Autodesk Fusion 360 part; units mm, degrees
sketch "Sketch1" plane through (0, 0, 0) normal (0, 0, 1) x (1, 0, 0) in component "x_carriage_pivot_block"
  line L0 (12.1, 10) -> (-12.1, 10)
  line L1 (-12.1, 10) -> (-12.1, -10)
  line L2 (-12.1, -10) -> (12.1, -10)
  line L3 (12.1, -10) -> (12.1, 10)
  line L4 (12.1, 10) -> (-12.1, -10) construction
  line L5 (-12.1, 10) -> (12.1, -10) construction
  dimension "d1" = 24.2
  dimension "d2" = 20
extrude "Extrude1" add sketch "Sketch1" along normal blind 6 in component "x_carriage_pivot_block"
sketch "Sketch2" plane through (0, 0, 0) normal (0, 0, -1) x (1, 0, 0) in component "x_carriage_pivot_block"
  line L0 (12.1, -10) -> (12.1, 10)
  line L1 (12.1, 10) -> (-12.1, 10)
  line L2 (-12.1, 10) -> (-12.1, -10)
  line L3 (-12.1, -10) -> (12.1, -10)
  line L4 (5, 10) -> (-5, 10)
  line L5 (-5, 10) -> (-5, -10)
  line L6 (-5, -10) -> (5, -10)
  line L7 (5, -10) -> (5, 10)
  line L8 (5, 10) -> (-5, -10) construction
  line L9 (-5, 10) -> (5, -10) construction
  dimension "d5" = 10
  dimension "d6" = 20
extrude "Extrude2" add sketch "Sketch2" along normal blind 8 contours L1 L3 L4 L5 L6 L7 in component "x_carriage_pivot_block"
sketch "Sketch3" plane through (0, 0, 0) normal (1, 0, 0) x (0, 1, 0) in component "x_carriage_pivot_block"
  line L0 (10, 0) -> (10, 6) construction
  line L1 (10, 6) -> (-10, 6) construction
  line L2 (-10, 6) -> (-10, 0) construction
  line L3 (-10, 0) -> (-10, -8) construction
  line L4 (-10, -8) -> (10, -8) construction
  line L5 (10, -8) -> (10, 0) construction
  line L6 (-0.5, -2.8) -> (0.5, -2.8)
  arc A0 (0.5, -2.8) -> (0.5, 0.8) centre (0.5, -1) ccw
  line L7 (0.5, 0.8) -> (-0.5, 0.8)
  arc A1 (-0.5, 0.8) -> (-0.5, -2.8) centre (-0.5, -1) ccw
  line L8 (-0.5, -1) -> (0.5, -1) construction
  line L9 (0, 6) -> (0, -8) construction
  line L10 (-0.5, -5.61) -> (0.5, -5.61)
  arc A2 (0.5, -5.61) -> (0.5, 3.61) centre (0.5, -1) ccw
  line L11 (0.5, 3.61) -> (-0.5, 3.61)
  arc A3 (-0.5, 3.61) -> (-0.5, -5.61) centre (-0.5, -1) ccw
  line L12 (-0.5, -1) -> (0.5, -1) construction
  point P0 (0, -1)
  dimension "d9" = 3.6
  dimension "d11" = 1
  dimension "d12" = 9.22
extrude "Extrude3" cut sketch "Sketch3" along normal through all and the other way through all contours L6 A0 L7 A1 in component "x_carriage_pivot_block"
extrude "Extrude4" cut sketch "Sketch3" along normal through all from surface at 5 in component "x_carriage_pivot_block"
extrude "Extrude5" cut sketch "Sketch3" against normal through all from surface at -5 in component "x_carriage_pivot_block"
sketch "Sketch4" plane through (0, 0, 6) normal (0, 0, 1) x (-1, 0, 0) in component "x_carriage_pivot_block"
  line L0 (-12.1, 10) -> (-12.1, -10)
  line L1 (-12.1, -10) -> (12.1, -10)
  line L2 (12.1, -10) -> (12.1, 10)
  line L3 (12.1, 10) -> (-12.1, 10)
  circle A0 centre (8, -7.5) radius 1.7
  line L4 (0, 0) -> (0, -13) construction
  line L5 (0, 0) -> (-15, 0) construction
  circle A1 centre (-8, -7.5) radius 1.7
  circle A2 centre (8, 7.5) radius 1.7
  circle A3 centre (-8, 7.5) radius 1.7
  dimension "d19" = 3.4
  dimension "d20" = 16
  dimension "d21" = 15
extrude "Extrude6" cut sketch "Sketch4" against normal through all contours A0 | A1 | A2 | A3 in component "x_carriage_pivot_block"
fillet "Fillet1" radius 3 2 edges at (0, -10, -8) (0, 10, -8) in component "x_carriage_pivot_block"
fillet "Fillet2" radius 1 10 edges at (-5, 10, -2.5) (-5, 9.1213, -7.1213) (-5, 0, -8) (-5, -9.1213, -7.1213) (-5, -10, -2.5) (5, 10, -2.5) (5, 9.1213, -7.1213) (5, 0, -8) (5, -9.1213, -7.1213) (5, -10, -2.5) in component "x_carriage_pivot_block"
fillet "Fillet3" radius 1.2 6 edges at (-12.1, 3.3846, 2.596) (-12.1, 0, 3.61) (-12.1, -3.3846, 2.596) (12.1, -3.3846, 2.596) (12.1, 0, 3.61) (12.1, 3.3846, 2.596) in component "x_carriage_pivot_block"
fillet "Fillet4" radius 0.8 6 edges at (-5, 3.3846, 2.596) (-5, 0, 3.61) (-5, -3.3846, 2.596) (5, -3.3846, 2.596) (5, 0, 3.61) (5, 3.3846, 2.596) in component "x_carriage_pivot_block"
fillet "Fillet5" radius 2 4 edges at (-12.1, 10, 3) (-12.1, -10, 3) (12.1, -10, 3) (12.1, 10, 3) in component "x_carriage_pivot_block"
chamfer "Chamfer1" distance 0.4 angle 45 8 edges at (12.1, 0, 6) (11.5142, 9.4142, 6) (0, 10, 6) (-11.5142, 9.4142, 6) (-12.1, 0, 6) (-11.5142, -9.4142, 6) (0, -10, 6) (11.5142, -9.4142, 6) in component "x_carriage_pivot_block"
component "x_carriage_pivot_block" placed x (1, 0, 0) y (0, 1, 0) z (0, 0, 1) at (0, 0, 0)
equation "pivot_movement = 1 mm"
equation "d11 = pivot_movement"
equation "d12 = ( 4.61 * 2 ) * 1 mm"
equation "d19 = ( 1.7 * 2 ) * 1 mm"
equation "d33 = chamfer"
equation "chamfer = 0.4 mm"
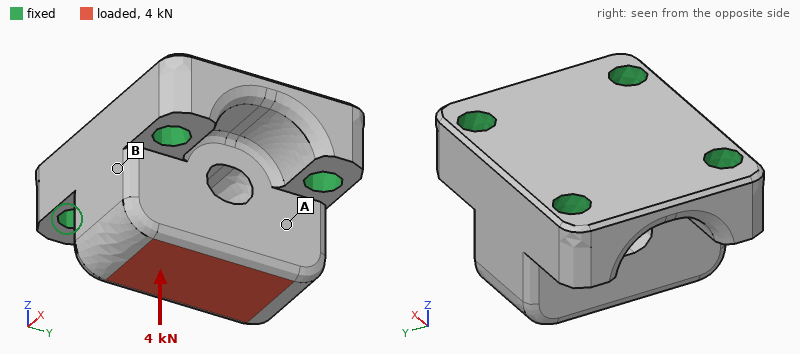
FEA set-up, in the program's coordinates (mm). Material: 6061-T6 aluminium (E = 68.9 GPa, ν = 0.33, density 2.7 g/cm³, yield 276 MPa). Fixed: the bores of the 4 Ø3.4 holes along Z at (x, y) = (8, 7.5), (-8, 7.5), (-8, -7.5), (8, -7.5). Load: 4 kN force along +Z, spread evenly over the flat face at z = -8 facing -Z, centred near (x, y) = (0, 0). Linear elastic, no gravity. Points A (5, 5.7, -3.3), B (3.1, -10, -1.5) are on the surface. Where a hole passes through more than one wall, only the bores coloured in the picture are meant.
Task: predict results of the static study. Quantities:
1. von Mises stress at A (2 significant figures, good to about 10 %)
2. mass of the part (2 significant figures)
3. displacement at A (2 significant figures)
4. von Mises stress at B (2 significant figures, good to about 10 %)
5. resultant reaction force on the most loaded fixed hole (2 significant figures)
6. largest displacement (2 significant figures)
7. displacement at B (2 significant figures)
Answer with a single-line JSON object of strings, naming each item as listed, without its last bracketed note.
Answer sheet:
{"von Mises stress at A": "28 MPa", "mass of the part": "9.9 g", "displacement at A": "5.8 µm", "von Mises stress at B": "14 MPa", "resultant reaction force on the most loaded fixed hole": "1.0 kN", "largest displacement": "10 µm", "displacement at B": "4.4 µm"}
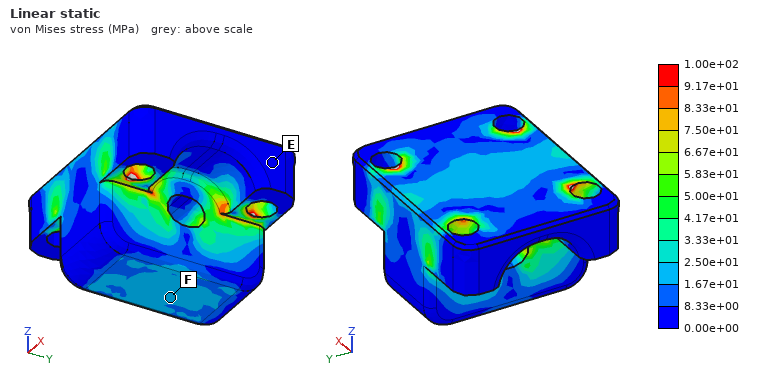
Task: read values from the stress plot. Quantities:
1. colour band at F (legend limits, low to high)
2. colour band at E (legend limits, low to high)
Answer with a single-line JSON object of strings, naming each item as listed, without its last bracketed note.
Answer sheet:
{"colour band at F": "1.67e+01 to 2.50e+01 MPa", "colour band at E": "0.00e+00 to 8.33e+00 MPa"}
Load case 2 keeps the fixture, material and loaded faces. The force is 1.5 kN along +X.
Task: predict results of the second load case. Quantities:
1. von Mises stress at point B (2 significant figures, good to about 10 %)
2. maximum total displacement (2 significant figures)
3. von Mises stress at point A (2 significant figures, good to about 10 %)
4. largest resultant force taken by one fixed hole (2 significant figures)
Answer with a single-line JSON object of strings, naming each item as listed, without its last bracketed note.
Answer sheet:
{"von Mises stress at point B": "19 MPa", "maximum total displacement": "14 µm", "von Mises stress at point A": "29 MPa", "largest resultant force taken by one fixed hole": "730 N"}
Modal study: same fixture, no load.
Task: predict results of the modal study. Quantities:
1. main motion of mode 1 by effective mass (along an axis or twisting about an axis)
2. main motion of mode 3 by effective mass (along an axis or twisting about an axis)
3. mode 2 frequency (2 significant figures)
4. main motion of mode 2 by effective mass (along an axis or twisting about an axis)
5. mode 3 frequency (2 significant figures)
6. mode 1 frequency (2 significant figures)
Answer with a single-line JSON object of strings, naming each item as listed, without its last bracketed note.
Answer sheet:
{"main motion of mode 1 by effective mass": "along Y", "main motion of mode 3 by effective mass": "along Z", "mode 2 frequency": "43 kHz", "main motion of mode 2 by effective mass": "along X", "mode 3 frequency": "53 kHz", "mode 1 frequency": "39 kHz"}
